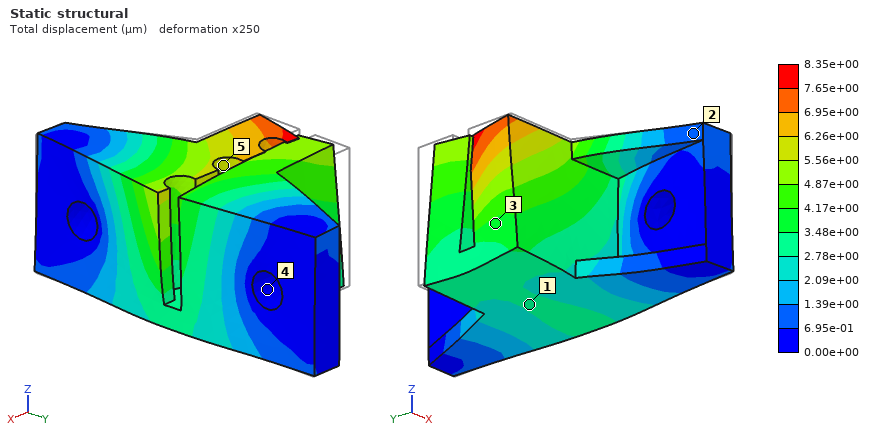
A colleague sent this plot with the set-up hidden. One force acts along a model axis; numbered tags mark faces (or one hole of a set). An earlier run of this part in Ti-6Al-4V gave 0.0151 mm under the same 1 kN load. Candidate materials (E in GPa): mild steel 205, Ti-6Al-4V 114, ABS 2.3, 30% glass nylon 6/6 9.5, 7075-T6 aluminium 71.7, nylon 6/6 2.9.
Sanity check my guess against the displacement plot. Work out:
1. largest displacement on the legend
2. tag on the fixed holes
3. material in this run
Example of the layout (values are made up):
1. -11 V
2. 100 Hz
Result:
1. 8.35e+00 µm
2. 4
3. mild steel
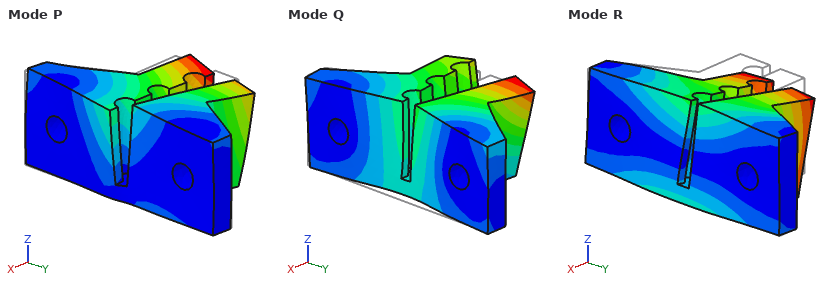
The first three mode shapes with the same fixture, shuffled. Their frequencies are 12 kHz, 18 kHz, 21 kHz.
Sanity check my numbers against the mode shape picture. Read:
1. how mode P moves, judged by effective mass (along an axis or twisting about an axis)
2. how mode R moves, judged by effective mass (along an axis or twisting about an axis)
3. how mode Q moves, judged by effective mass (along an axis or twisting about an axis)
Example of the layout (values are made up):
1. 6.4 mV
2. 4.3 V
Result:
1. along Y
2. along Z
3. along X
